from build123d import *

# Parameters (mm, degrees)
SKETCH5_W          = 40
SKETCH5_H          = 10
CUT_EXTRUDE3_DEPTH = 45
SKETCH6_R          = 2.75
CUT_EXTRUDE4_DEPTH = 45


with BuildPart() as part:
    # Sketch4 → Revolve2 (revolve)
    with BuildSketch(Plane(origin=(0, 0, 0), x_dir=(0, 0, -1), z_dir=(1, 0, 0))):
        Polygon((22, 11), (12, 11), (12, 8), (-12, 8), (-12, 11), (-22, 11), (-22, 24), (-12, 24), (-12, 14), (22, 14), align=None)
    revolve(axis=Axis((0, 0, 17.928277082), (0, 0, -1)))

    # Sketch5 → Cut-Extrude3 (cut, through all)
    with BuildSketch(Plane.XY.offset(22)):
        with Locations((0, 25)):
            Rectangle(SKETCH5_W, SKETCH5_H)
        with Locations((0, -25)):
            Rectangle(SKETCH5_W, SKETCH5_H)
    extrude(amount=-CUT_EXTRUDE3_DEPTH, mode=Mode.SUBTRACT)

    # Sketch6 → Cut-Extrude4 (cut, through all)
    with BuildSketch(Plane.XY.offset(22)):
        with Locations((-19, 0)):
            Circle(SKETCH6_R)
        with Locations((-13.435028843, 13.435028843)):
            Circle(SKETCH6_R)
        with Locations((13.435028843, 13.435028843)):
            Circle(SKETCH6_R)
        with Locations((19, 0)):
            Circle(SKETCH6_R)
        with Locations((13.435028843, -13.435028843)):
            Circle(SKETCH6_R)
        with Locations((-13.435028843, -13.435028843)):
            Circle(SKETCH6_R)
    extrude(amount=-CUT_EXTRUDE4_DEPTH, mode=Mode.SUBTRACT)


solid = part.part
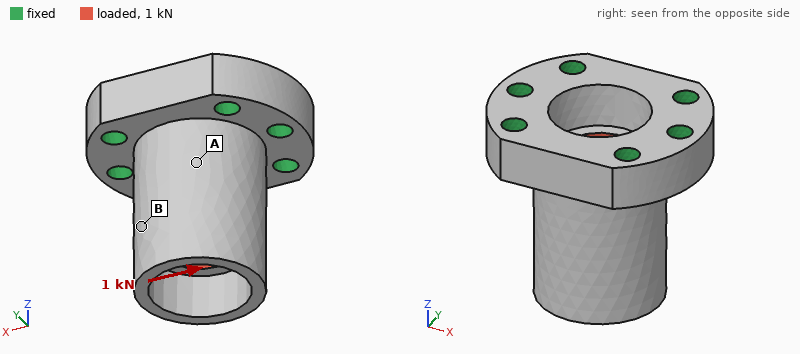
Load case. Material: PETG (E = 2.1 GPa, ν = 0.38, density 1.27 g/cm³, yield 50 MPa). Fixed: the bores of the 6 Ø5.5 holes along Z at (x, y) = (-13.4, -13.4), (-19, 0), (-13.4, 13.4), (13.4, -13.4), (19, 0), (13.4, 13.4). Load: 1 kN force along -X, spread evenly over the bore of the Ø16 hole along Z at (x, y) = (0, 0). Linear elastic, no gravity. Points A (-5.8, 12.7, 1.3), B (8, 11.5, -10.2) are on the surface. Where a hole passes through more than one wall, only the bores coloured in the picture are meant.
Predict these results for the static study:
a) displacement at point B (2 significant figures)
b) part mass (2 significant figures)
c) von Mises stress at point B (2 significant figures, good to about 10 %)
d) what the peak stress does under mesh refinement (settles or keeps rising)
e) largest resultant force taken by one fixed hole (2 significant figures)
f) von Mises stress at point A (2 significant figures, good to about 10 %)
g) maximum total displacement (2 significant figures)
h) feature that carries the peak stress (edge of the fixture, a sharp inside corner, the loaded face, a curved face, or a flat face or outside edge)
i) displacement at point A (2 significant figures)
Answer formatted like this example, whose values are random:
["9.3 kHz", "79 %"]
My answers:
["0.12 mm", "30 g", "1.1 MPa", "keeps rising", "320 N", "3.1 MPa", "0.16 mm", "a sharp inside corner", "0.072 mm"]
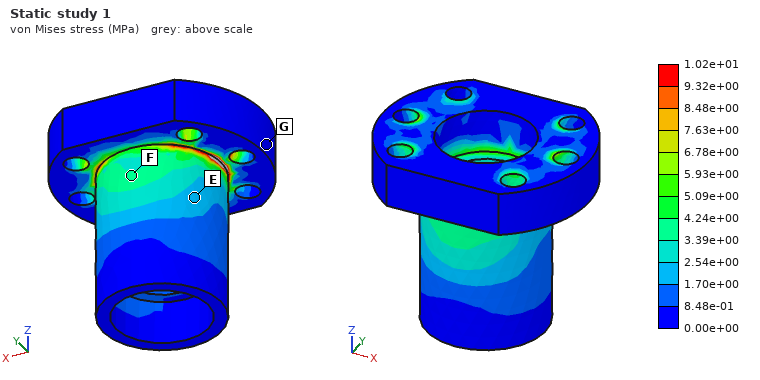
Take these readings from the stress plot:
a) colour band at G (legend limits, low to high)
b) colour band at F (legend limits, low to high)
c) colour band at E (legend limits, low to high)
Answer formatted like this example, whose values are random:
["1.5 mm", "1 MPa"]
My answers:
["0.00e+00 to 8.48e-01 MPa", "3.39e+00 to 4.24e+00 MPa", "1.70e+00 to 2.54e+00 MPa"]
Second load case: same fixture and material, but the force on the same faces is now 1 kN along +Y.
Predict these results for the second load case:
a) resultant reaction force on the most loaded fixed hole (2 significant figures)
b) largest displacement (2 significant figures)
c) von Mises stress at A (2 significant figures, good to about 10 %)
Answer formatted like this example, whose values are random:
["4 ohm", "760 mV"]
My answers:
["370 N", "0.20 mm", "2.1 MPa"]
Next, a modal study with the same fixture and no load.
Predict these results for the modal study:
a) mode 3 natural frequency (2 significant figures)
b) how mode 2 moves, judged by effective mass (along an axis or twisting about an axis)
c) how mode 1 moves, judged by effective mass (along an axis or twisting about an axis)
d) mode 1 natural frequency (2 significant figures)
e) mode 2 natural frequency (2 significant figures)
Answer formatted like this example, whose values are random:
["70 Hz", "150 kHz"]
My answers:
["5300 Hz", "along X", "along Y", "2900 Hz", "3200 Hz"]
